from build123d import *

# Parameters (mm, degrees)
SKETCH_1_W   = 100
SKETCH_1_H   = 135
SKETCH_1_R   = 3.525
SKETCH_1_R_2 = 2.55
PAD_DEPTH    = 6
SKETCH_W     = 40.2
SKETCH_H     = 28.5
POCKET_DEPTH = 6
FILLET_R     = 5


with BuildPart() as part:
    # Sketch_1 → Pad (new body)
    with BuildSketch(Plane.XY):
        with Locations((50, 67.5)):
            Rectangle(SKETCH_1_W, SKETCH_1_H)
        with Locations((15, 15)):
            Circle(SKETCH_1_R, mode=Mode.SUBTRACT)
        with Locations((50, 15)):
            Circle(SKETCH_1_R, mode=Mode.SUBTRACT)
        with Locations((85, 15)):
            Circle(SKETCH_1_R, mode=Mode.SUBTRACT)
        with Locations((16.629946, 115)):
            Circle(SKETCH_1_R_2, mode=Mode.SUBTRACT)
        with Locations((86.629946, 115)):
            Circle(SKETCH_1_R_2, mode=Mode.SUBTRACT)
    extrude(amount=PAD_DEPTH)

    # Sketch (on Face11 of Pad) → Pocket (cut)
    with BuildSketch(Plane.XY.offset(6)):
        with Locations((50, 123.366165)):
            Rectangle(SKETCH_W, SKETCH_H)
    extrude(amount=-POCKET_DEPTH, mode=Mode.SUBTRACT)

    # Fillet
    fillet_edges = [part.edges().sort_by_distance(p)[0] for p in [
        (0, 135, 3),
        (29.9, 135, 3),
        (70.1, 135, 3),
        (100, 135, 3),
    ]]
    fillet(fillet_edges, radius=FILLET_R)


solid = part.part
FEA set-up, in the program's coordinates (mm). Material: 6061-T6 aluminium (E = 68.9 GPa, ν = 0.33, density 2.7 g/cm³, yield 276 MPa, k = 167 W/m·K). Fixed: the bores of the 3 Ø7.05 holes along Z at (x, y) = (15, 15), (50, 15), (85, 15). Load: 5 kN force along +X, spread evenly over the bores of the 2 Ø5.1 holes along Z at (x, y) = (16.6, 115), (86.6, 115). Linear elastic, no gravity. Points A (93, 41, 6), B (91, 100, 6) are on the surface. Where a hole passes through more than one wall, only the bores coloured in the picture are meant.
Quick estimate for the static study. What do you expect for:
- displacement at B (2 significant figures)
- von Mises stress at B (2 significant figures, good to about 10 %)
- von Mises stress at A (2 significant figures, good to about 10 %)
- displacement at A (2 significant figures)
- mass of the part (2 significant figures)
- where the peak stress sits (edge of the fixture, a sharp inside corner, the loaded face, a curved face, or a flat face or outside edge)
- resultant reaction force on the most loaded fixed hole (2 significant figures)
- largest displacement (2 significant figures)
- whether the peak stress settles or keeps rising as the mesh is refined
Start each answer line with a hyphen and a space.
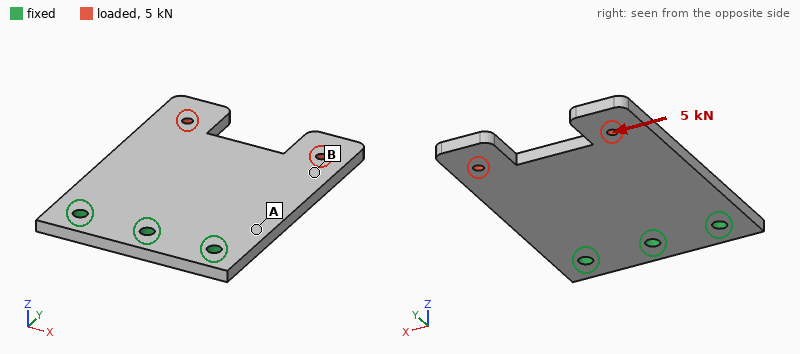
- 0.090 mm
- 15 MPa
- 32 MPa
- 0.027 mm
- 200 g
- edge of the fixture
- 7.0 kN
- 0.14 mm
- keeps rising
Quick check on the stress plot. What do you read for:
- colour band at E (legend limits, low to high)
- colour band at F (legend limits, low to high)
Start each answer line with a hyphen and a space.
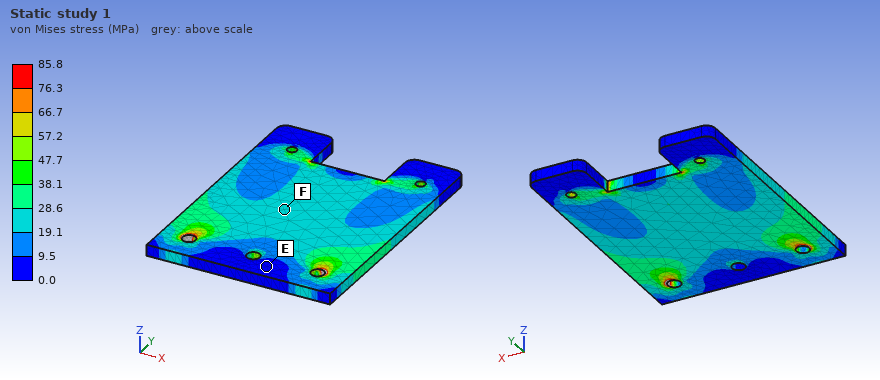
- 0.0 to 9.5 MPa
- 19.1 to 28.6 MPa
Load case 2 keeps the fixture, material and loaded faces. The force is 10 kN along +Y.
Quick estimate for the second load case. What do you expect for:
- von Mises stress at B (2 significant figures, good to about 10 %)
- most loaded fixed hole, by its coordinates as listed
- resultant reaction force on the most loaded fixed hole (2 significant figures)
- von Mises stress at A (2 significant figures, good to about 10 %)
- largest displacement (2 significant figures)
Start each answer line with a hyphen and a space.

- 34 MPa
- (85, 15)
- 3.7 kN
- 19 MPa
- 47 µm
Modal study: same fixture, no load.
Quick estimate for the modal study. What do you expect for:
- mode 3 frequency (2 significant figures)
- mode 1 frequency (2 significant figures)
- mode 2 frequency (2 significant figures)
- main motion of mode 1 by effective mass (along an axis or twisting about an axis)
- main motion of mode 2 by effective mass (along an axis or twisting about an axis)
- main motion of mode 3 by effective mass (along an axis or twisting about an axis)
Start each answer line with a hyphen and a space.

- 2300 Hz
- 410 Hz
- 900 Hz
- along Z
- twisting about Y
- along Z
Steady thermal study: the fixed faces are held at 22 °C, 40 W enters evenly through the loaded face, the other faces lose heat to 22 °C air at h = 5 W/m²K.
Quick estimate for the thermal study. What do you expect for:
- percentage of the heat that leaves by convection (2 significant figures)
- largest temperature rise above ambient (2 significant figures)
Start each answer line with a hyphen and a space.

- 6.8 %
- 47 K
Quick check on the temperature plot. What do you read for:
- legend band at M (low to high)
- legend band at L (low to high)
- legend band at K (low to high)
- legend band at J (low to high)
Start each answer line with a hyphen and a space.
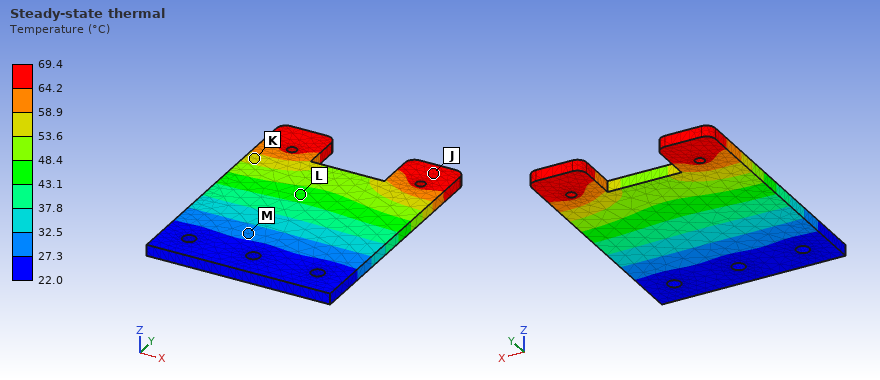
- 27.3 to 32.5 °C
- 43.1 to 48.4 °C
- 53.6 to 58.9 °C
- 64.2 to 69.4 °C
